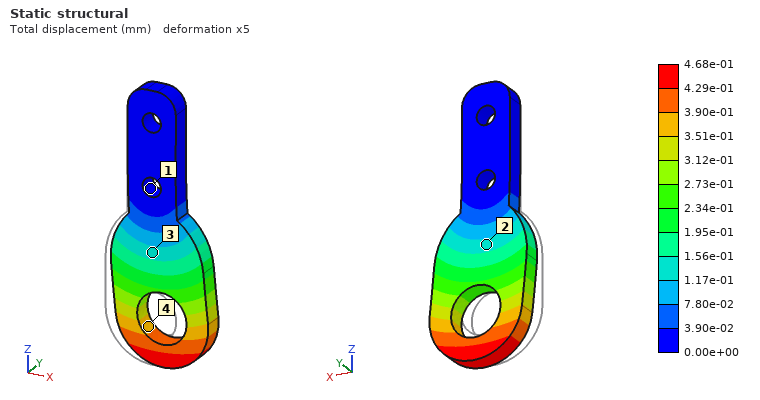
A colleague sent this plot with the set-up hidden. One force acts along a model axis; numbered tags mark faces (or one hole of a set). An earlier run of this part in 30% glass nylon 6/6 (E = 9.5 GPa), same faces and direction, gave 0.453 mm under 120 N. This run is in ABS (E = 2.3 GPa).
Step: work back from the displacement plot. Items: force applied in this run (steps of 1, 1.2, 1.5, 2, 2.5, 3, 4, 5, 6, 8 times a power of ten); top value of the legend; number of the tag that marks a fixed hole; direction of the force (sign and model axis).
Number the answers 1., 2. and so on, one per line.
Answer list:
1. 30 N
2. 4.68e-01 mm
3. 1
4. +X
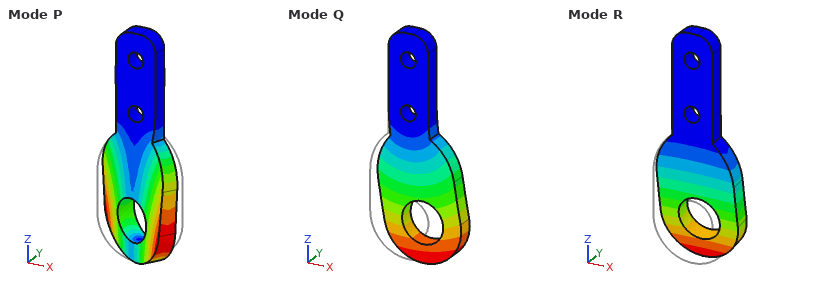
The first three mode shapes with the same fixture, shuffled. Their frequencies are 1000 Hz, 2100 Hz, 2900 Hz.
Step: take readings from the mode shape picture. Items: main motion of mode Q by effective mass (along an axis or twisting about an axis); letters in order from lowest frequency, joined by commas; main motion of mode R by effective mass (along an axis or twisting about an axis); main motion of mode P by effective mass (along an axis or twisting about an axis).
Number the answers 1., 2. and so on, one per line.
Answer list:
1. along X
2. R, Q, P
3. along Y
4. twisting about Z
